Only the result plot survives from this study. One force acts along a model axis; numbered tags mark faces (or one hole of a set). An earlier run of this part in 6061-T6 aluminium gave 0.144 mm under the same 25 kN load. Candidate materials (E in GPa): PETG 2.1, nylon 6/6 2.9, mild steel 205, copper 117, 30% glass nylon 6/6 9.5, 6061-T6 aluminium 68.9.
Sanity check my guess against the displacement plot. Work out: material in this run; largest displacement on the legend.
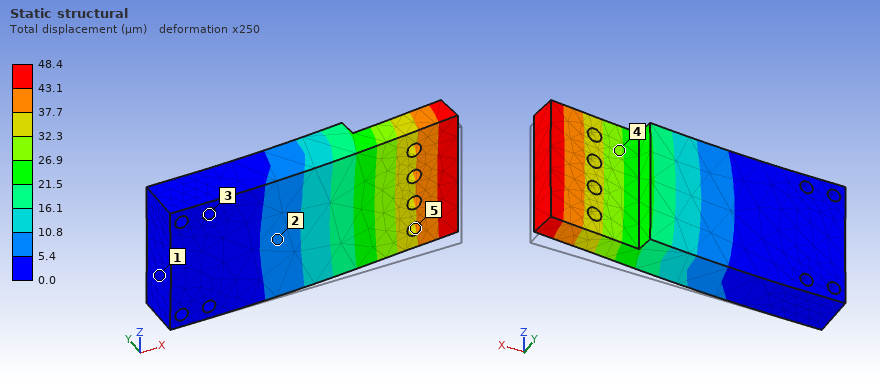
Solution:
mild steel
48.4 µm
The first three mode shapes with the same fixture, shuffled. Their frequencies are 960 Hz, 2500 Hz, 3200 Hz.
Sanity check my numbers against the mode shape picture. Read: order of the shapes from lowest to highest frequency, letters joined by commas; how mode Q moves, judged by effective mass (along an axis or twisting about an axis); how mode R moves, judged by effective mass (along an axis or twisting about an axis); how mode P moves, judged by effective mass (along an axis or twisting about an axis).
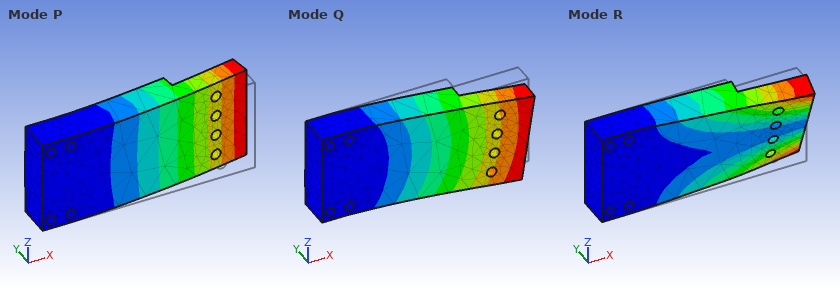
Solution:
P, Q, R
along Z
twisting about X
along Y
